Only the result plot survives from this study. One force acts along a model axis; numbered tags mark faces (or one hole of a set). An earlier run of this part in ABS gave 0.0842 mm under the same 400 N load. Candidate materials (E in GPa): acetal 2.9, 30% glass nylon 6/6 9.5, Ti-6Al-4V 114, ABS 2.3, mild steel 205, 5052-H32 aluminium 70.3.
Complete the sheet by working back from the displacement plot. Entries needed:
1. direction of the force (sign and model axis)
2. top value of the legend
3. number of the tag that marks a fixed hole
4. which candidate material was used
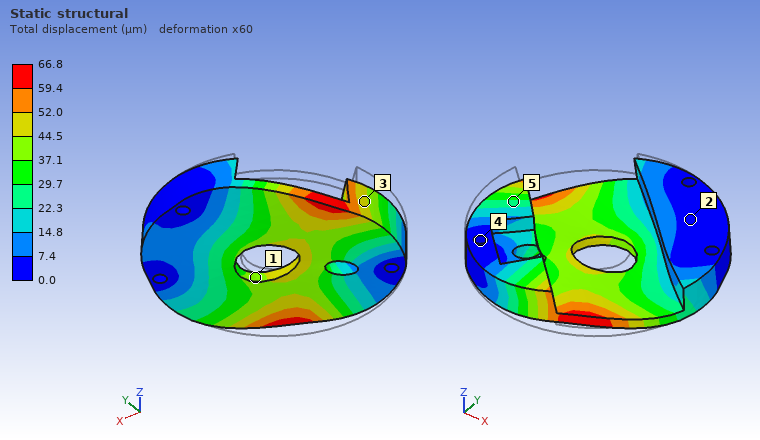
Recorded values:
+X
66.8 µm
4
acetal
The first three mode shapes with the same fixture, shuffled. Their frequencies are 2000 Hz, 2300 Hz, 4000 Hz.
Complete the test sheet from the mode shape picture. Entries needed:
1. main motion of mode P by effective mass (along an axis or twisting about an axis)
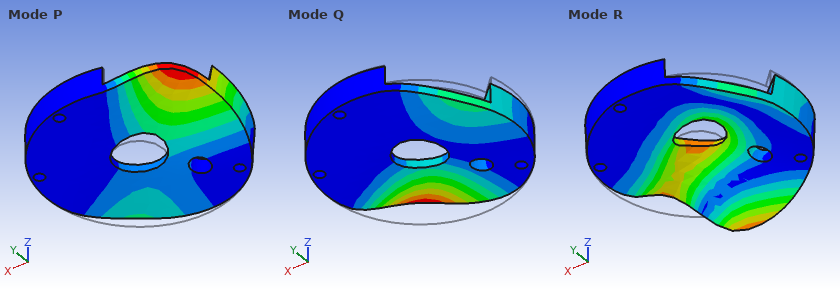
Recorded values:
along Z
